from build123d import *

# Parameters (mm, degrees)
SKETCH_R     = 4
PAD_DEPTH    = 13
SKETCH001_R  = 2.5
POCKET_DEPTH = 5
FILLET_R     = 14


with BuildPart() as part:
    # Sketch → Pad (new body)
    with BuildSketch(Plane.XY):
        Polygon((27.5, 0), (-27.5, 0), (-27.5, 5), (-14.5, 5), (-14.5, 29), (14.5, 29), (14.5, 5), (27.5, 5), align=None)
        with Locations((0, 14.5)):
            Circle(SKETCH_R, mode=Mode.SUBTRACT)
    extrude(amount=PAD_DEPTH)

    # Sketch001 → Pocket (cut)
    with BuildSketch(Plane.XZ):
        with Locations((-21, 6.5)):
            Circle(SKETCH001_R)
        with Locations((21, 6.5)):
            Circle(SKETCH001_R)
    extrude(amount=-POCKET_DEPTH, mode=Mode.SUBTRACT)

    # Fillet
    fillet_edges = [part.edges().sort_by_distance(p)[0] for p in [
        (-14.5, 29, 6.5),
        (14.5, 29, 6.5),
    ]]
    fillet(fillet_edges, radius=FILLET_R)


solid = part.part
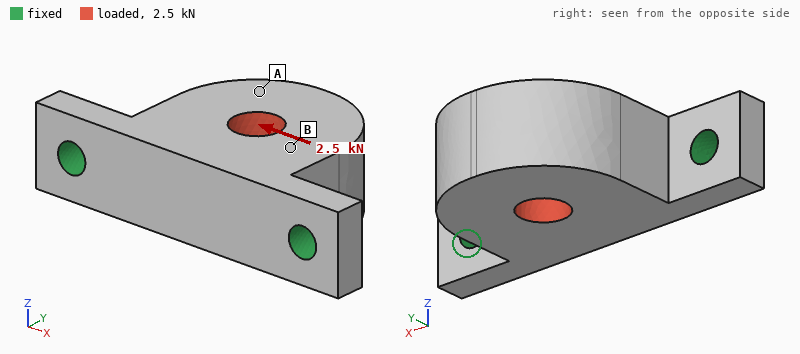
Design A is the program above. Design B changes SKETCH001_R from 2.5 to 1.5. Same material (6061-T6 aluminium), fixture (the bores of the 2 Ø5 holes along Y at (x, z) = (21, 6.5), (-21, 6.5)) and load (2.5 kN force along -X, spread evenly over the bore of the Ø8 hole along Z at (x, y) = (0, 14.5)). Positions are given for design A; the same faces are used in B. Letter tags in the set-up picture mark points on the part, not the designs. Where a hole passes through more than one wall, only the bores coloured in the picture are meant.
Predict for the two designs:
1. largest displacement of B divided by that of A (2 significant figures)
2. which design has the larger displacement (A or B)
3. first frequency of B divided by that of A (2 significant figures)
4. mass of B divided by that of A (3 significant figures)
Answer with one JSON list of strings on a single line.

["1.2", "B", "0.87", "1.01"]
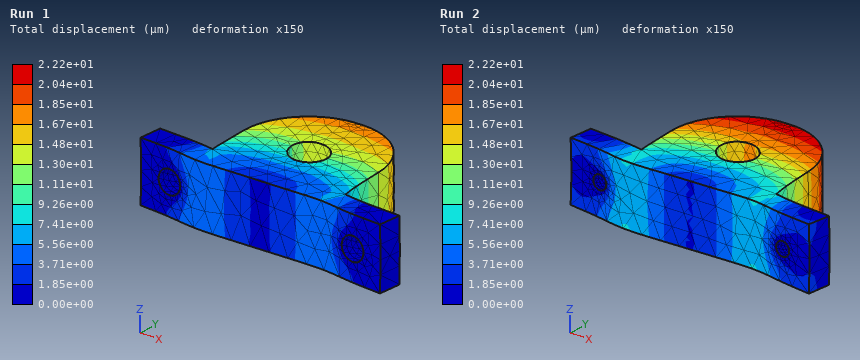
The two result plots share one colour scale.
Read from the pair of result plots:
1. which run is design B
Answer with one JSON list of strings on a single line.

["Run 2"]
